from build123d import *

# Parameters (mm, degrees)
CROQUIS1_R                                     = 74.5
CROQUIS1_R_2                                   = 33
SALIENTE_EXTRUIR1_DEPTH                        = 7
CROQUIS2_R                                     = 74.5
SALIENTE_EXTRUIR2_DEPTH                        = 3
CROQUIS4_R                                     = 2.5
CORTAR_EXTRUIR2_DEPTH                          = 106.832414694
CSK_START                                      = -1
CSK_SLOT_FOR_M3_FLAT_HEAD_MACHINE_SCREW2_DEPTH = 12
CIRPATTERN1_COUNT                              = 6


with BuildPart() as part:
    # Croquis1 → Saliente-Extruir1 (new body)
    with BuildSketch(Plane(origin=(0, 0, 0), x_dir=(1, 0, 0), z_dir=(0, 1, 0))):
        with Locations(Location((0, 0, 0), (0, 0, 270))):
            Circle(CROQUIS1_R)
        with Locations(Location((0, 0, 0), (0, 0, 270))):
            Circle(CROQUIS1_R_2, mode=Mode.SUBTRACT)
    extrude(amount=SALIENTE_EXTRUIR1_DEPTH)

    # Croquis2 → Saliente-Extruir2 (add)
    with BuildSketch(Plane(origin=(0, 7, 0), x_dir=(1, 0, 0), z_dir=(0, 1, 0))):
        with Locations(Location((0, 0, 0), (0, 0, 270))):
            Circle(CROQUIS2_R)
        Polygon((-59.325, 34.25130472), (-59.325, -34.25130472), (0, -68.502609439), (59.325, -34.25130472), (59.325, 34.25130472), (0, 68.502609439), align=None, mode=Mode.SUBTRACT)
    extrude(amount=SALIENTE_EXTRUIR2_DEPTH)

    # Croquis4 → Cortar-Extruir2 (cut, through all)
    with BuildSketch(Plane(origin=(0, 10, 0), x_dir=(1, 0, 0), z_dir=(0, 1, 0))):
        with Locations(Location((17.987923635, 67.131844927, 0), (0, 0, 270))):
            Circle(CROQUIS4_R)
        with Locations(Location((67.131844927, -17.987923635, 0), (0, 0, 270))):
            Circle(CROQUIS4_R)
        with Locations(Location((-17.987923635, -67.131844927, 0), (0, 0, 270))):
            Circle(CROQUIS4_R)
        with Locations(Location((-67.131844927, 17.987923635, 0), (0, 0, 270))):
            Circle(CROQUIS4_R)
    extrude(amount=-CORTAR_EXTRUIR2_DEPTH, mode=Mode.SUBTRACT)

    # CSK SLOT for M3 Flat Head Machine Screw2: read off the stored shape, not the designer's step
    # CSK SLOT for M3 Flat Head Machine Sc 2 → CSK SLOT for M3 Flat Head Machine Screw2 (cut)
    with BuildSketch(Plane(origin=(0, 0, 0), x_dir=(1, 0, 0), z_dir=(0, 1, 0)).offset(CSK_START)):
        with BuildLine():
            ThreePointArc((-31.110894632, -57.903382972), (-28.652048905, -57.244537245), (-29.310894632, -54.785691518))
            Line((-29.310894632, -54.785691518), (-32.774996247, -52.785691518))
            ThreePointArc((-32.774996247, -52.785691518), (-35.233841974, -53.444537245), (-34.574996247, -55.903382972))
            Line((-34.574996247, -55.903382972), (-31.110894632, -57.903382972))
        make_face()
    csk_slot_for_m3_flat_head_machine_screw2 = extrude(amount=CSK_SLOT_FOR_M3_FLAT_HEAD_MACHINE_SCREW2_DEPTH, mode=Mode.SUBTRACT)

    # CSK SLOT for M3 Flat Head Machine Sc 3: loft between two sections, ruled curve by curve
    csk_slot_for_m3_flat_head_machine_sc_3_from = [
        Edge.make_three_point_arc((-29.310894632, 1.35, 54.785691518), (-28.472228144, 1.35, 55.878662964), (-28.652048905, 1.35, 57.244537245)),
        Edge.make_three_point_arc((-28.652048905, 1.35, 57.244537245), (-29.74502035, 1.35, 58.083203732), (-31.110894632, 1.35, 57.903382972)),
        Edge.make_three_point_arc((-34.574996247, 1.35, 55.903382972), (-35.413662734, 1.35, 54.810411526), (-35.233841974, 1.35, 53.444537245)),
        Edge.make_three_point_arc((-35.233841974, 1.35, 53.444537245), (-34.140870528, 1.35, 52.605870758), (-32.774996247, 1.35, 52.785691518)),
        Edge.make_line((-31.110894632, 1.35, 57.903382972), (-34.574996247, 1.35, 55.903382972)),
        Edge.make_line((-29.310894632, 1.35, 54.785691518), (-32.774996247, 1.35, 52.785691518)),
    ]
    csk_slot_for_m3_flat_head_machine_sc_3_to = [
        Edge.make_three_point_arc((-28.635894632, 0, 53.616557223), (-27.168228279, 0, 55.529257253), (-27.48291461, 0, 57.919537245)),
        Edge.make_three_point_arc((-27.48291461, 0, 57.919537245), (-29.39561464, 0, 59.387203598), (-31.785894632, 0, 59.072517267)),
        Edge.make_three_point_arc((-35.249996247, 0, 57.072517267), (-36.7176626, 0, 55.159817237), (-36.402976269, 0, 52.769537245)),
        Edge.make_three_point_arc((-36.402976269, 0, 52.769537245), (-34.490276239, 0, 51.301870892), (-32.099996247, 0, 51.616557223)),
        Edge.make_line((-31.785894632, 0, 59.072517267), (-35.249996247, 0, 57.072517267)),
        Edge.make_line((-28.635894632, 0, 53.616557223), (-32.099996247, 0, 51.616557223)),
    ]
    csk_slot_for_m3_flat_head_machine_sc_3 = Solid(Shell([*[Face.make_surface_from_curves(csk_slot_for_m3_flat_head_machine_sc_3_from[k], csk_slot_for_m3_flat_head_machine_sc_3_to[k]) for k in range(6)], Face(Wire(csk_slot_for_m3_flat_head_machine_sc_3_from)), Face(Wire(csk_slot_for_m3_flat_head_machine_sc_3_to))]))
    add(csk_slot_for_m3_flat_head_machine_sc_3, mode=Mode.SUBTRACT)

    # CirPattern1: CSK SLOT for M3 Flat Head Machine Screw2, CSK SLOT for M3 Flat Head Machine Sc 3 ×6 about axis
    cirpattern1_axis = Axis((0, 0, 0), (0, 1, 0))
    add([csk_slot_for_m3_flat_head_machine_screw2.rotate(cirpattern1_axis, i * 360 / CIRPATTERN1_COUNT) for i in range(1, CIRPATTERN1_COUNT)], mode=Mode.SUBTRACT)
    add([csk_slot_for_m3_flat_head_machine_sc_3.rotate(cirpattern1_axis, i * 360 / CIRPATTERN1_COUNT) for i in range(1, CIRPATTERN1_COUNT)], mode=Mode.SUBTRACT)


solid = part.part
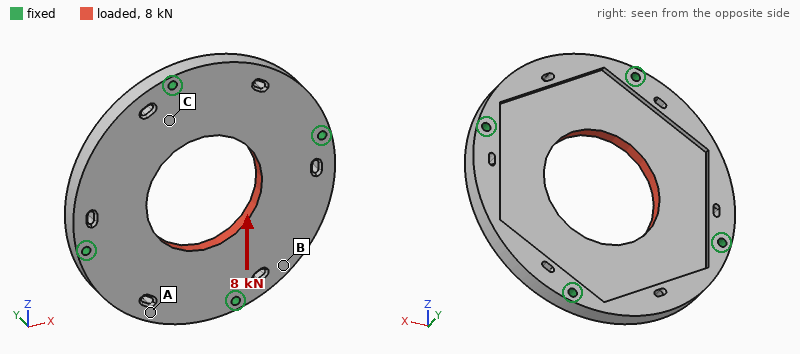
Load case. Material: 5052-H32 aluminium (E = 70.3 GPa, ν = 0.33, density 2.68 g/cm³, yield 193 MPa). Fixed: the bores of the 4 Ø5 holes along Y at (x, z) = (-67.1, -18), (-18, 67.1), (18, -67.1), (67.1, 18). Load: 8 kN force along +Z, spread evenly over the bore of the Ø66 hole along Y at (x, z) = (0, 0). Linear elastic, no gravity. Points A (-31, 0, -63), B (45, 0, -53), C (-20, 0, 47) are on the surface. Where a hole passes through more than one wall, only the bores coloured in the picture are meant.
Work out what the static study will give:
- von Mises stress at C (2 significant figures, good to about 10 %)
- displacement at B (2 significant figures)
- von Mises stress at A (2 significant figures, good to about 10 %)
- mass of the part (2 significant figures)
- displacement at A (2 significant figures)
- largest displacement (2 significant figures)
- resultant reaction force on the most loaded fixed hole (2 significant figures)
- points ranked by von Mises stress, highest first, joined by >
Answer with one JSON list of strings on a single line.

["11 MPa", "4.9 µm", "6.5 MPa", "300 g", "7.3 µm", "9.7 µm", "2.1 kN", "C > A > B"]
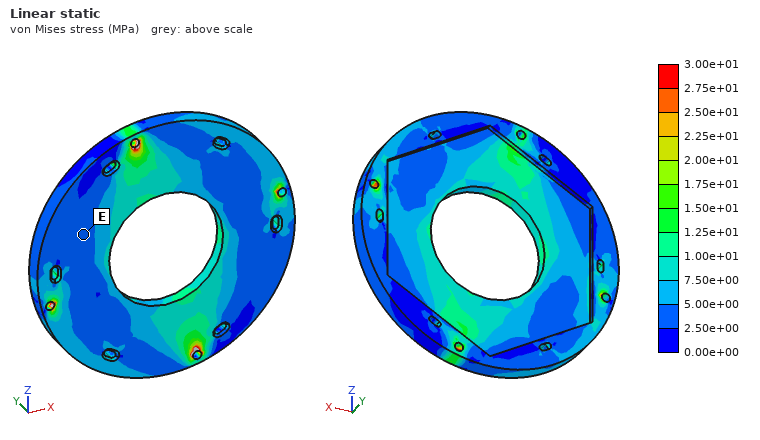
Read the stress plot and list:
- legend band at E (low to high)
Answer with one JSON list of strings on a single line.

["2.50e+00 to 5.00e+00 MPa"]
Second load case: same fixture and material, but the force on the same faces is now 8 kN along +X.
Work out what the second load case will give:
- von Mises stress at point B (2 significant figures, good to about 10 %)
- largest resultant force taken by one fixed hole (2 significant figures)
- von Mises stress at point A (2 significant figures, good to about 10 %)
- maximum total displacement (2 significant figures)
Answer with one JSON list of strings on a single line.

["5.7 MPa", "2.1 kN", "4.2 MPa", "9.8 µm"]
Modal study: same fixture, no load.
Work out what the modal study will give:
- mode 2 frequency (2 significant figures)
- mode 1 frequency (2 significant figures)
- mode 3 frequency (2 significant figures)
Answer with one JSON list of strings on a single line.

["3800 Hz", "3700 Hz", "3900 Hz"]
